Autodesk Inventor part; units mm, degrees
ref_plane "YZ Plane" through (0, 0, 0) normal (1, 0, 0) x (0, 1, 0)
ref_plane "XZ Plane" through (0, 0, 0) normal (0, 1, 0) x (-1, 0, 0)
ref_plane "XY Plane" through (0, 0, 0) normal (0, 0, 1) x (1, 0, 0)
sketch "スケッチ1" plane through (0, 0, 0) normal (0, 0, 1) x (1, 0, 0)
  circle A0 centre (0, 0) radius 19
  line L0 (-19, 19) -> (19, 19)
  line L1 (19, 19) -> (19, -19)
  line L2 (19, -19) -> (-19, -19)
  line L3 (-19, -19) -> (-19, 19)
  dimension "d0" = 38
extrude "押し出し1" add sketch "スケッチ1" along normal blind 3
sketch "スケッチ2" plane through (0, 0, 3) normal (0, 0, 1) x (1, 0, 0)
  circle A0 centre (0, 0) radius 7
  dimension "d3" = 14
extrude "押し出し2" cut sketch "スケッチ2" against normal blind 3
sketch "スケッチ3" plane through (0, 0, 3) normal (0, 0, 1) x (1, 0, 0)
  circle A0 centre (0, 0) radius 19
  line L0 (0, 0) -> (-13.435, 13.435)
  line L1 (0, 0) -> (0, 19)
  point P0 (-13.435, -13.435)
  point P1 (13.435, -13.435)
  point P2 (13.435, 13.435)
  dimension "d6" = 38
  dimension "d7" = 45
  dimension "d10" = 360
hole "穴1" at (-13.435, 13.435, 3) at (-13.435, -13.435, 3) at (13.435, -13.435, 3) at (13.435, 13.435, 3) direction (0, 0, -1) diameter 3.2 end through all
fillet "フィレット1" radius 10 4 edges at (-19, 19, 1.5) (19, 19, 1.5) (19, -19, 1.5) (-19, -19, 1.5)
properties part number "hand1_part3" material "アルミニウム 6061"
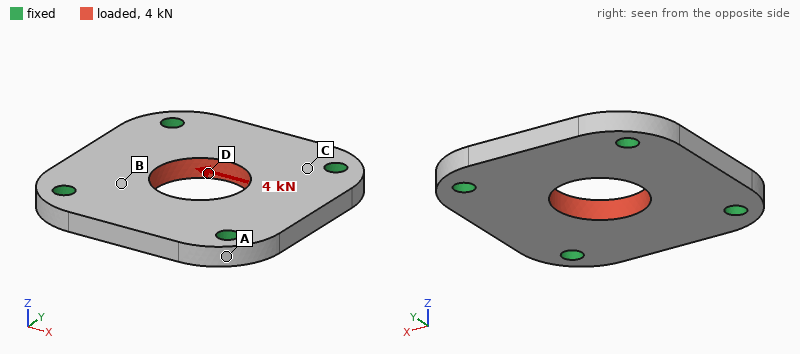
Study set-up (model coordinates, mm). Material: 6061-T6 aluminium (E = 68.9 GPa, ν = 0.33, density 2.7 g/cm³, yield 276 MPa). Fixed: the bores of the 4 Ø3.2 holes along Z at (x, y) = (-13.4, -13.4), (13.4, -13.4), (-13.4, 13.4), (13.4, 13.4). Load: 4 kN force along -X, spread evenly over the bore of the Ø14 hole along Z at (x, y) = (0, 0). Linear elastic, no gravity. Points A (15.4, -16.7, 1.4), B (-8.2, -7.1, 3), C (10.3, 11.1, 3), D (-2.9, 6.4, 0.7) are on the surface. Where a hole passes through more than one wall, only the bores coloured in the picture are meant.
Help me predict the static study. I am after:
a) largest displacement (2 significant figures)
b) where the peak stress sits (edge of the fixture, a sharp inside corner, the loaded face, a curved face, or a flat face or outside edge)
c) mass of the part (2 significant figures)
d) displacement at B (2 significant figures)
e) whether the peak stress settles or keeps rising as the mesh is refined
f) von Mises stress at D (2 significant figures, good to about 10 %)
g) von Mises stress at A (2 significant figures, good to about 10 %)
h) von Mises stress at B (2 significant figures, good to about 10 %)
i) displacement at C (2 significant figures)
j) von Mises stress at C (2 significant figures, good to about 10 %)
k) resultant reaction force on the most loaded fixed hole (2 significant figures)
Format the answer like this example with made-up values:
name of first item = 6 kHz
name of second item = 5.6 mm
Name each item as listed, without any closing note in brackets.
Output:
largest displacement = 11 µm
where the peak stress sits = edge of the fixture
mass of the part = 9.5 g
displacement at B = 6.1 µm
whether the peak stress settles or keeps rising as the mesh is refined = keeps rising
von Mises stress at D = 55 MPa
von Mises stress at A = 21 MPa
von Mises stress at B = 33 MPa
displacement at C = 2.3 µm
von Mises stress at C = 48 MPa
resultant reaction force on the most loaded fixed hole = 1.1 kN
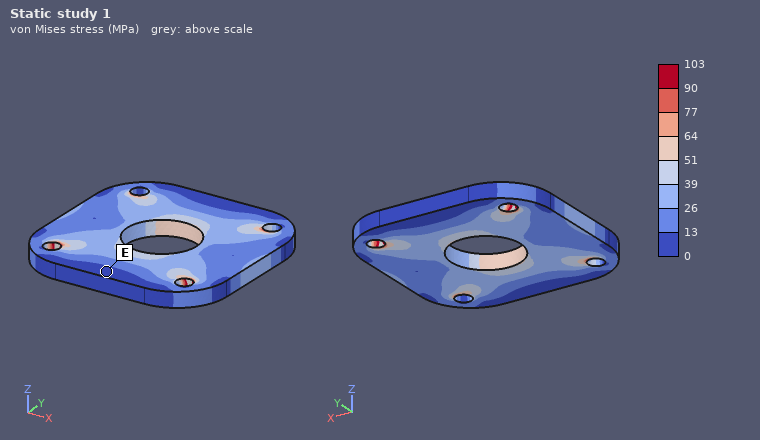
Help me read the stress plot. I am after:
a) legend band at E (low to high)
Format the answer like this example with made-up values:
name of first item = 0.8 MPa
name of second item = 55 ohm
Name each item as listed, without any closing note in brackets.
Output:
legend band at E = 0 to 13 MPa
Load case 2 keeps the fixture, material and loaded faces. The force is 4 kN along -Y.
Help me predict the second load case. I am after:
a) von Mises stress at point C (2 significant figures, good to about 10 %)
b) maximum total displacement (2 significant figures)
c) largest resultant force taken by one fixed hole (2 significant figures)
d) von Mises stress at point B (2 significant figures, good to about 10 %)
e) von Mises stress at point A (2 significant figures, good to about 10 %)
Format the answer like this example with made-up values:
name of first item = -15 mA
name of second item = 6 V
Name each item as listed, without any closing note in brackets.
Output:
von Mises stress at point C = 46 MPa
maximum total displacement = 11 µm
largest resultant force taken by one fixed hole = 1.1 kN
von Mises stress at point B = 34 MPa
von Mises stress at point A = 25 MPa
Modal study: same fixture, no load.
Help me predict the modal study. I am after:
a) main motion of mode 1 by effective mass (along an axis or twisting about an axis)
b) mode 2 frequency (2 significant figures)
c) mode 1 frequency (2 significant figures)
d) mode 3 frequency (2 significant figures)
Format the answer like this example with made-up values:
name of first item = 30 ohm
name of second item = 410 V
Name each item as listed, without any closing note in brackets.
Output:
main motion of mode 1 by effective mass = along Z
mode 2 frequency = 22 kHz
mode 1 frequency = 18 kHz
mode 3 frequency = 22 kHz
